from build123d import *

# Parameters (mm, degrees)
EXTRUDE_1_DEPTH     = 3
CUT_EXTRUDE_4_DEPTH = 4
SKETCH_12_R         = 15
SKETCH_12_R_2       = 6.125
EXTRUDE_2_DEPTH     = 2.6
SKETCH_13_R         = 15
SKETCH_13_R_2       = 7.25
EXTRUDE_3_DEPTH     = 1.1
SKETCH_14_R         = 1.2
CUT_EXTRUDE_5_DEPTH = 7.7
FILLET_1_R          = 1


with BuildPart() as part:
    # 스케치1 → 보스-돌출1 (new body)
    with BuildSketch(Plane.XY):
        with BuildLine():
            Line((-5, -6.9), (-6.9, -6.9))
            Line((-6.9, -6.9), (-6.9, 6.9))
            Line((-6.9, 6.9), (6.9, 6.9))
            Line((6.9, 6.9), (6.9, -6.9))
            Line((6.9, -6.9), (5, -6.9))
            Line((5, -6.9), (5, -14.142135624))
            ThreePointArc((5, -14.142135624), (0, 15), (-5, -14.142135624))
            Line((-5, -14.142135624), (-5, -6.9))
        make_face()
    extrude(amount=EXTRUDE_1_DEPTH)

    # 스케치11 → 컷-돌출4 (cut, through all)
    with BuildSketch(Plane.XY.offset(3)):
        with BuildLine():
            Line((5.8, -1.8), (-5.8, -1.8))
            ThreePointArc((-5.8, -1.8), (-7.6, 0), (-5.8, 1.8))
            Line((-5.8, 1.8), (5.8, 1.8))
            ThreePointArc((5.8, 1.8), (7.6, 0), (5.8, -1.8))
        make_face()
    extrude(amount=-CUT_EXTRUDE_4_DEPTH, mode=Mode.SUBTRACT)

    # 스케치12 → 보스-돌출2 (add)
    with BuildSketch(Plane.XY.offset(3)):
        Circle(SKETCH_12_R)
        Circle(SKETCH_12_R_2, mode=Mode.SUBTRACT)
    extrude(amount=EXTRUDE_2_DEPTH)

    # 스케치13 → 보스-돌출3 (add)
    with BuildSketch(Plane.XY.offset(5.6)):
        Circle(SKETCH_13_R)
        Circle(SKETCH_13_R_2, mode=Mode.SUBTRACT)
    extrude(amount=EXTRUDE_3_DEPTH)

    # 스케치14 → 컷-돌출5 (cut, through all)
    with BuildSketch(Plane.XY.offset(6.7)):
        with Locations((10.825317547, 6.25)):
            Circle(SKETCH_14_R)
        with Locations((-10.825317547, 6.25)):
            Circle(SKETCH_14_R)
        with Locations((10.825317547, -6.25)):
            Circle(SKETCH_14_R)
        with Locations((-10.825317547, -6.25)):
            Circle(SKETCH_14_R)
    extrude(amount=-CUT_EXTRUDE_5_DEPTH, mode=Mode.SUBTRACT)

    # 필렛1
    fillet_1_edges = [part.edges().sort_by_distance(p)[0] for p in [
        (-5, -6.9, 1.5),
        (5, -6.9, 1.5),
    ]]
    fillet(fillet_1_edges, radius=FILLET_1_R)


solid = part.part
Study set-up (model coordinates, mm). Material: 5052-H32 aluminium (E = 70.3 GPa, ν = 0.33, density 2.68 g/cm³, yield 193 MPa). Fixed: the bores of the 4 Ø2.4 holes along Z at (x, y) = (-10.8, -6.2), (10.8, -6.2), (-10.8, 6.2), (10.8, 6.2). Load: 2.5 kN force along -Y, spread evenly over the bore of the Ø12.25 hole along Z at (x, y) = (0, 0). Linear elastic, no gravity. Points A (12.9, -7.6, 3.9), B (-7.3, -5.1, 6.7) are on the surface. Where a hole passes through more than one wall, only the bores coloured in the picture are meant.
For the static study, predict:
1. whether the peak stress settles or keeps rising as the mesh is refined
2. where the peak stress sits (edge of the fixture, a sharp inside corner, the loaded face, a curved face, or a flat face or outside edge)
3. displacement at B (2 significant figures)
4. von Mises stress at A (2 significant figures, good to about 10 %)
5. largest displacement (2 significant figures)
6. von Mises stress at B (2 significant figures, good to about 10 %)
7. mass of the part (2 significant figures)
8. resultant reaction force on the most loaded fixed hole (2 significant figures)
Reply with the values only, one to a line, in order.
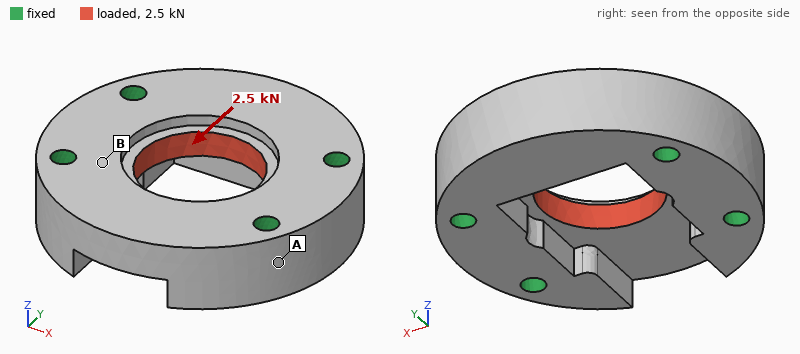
keeps rising
edge of the fixture
1.7 µm
6.6 MPa
5.8 µm
16 MPa
8.9 g
640 N
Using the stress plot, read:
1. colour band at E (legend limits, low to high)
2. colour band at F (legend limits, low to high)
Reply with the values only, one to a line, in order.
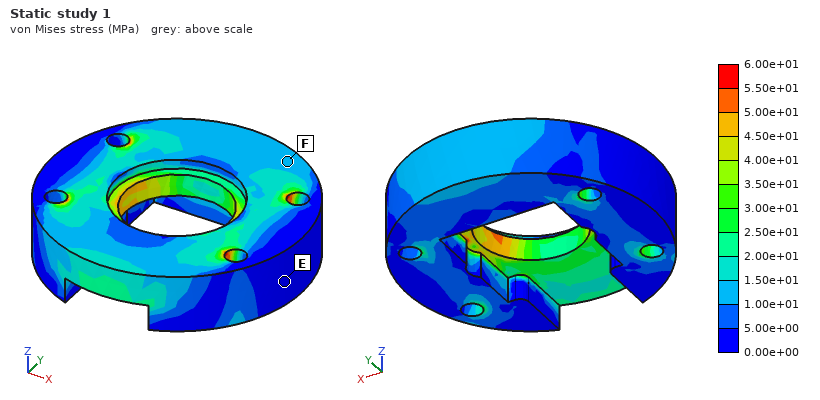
0.00e+00 to 5.00e+00 MPa
1.00e+01 to 1.50e+01 MPa
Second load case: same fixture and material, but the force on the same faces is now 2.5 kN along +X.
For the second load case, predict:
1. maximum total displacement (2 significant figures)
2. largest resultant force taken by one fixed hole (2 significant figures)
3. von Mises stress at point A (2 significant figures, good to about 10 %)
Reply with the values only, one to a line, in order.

3.0 µm
640 N
8.7 MPa
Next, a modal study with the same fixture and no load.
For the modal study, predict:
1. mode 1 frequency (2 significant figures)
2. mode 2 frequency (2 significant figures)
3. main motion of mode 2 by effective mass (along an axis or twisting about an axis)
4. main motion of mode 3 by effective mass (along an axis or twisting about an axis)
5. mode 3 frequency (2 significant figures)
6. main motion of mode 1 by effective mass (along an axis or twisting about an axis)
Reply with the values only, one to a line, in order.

37 kHz
41 kHz
along Z
along Y
62 kHz
along Z
